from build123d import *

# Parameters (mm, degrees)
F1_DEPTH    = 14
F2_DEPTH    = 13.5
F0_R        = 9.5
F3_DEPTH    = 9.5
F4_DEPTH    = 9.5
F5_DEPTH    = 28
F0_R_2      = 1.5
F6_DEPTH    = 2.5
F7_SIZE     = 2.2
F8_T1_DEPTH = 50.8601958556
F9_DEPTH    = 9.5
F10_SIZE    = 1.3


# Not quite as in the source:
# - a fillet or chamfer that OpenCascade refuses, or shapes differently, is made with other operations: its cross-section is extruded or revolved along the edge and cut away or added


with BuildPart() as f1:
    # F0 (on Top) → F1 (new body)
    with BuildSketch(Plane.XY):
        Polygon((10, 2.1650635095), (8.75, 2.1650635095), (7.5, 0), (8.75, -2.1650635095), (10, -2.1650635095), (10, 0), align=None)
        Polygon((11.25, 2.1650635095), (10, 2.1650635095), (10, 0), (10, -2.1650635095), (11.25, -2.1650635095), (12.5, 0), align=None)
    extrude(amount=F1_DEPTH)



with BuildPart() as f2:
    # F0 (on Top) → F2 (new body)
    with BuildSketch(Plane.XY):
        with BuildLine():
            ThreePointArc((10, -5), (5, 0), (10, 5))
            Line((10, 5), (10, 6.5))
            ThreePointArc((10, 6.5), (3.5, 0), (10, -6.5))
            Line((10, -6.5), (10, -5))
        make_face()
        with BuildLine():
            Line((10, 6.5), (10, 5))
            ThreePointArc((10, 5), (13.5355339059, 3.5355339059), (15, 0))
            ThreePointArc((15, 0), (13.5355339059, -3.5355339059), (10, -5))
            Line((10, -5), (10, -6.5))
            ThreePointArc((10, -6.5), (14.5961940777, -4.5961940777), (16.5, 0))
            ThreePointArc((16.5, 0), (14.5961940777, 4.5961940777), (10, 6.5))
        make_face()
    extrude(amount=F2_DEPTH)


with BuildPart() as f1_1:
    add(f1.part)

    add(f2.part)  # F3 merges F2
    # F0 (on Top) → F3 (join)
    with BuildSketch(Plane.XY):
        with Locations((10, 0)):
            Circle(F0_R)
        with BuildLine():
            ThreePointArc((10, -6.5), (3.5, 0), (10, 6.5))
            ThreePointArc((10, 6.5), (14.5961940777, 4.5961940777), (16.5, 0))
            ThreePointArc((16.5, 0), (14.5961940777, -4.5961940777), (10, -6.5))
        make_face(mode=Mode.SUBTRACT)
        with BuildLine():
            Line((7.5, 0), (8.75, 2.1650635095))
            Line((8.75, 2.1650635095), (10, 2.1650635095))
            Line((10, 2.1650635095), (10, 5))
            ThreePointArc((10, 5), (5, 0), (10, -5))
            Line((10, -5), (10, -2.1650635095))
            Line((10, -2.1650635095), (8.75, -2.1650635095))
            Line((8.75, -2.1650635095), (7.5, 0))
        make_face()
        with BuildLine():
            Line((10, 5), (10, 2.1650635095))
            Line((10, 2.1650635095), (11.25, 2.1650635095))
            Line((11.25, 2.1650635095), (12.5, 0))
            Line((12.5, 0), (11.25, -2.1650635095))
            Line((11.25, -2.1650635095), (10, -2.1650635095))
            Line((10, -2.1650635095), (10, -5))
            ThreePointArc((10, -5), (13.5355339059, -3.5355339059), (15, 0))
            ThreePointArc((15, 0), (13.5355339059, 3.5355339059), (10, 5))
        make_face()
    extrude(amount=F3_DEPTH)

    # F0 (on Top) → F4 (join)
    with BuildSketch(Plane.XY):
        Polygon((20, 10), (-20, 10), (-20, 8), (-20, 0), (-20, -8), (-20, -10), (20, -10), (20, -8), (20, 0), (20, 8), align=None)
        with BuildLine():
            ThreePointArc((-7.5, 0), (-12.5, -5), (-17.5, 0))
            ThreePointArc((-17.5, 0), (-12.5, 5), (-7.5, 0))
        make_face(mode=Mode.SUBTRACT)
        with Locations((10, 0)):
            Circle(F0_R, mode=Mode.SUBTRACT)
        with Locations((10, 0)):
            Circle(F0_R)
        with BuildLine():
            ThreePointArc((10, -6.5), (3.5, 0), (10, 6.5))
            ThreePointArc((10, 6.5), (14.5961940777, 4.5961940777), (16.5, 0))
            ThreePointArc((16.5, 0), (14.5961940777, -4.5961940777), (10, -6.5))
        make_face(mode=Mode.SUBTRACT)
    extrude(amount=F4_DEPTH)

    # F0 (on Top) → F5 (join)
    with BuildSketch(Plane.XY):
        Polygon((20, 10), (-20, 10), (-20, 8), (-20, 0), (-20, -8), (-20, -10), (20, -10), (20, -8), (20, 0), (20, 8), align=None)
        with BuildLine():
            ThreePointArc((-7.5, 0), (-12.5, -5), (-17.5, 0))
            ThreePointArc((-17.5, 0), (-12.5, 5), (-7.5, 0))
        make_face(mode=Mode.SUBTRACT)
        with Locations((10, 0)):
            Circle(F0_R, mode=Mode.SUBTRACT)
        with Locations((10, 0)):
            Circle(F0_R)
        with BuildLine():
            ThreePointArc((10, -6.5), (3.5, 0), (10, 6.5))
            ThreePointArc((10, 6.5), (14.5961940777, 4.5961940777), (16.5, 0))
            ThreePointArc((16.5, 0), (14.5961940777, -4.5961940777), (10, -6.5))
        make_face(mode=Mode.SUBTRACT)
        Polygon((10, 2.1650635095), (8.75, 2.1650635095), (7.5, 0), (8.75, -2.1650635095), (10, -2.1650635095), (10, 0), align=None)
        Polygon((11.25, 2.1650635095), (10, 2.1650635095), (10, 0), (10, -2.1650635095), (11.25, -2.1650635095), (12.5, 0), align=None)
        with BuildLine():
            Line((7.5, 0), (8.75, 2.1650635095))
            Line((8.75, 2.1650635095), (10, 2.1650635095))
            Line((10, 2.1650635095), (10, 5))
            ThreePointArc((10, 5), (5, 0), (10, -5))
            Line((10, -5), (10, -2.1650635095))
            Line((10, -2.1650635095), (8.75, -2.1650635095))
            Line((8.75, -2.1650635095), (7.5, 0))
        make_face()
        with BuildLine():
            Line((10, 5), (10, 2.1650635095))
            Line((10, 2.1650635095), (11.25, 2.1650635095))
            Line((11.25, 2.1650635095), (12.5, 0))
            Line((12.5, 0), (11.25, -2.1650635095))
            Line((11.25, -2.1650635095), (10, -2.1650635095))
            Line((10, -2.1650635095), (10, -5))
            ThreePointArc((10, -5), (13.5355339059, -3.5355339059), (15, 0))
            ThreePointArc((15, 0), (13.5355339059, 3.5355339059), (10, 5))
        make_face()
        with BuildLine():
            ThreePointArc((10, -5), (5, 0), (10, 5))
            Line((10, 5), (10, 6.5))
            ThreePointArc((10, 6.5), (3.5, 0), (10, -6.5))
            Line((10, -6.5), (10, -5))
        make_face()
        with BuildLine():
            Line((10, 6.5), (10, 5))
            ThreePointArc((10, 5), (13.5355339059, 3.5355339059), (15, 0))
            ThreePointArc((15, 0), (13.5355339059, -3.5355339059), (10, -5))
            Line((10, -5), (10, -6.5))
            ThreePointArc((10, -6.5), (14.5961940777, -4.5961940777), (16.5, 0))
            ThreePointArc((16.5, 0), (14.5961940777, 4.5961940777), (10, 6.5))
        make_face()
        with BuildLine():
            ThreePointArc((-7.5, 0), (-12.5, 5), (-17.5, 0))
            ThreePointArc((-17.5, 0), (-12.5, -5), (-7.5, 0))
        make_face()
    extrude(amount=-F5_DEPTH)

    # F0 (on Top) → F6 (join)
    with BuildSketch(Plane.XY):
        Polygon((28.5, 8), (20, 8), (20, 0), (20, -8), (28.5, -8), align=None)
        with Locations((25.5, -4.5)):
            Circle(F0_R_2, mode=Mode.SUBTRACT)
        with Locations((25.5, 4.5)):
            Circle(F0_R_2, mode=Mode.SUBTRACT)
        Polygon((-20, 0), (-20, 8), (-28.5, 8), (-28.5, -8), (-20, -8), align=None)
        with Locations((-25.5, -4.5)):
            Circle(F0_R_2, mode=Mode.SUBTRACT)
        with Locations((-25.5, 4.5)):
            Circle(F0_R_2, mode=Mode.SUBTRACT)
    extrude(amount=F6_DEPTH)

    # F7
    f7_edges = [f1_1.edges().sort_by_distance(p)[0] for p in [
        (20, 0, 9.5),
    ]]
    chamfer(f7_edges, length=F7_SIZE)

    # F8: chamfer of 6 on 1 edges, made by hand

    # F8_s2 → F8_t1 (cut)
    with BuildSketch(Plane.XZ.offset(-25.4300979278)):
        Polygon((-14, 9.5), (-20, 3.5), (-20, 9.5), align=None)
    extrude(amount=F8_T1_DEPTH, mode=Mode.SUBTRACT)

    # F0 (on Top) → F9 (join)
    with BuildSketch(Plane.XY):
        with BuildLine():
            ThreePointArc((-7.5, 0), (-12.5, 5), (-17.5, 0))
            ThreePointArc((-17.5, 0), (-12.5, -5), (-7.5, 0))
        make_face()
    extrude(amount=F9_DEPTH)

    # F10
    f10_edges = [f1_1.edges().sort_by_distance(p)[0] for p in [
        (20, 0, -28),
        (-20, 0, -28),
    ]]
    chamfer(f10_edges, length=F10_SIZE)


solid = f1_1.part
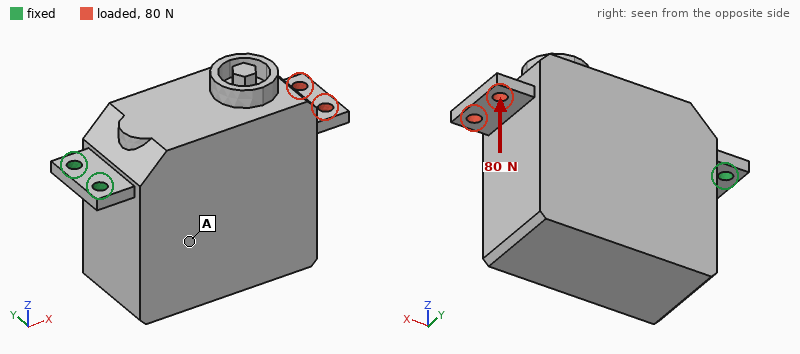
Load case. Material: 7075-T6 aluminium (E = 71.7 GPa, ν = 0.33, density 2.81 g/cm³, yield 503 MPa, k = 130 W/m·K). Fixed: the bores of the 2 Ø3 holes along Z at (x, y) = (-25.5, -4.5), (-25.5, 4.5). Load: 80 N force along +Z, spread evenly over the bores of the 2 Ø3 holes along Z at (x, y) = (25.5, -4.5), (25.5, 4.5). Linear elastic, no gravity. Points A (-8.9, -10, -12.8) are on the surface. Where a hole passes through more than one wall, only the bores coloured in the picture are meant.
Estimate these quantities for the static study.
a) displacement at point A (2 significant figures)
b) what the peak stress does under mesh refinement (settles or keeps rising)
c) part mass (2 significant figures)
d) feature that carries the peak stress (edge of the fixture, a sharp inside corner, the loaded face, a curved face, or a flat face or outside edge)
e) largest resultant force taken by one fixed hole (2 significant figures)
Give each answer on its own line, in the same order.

0.25 mm
keeps rising
86 g
edge of the fixture
41 N
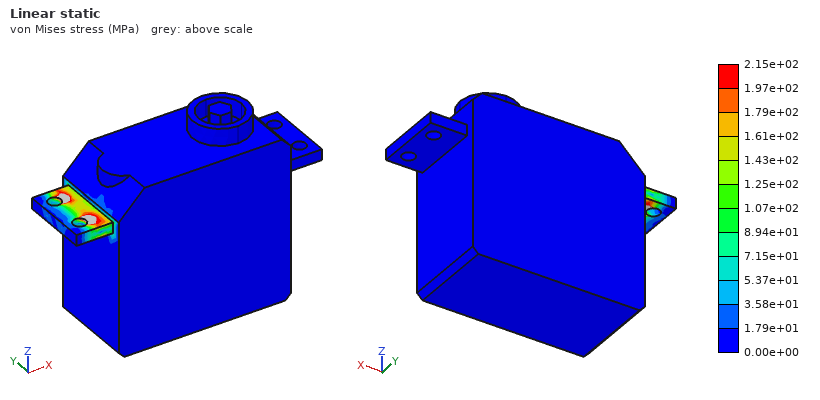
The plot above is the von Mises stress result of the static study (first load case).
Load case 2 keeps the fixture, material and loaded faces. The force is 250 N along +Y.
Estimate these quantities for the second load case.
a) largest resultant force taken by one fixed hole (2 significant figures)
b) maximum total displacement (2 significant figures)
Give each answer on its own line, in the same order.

1.2 kN
86 µm
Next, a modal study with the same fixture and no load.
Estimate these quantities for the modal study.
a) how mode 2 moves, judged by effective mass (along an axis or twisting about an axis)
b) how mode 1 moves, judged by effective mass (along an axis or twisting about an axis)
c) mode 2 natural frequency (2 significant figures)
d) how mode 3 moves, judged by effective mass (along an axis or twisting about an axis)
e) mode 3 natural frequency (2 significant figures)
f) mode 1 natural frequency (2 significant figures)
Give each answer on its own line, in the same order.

along Y
along Z
1300 Hz
along Y
2400 Hz
320 Hz
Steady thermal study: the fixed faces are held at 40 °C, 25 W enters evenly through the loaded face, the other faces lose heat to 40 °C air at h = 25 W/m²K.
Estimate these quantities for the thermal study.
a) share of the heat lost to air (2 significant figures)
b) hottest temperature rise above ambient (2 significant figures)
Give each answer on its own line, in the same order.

21 %
79 K
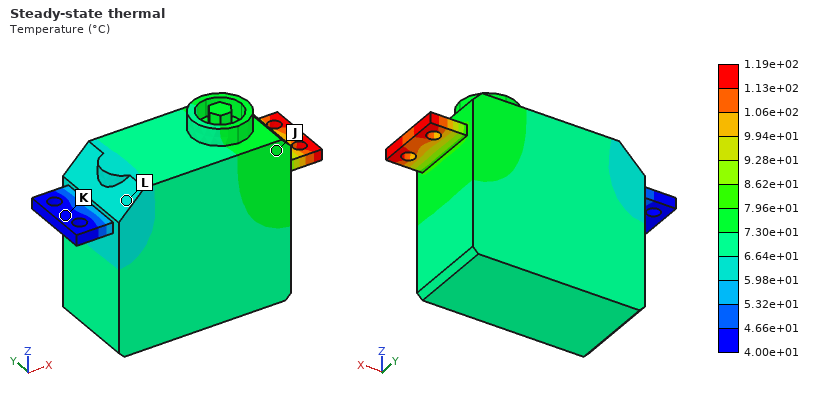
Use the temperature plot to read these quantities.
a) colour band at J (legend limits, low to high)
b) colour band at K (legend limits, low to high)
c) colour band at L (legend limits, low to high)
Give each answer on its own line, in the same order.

7.30e+01 to 7.96e+01 °C
4.00e+01 to 4.66e+01 °C
5.98e+01 to 6.64e+01 °C
